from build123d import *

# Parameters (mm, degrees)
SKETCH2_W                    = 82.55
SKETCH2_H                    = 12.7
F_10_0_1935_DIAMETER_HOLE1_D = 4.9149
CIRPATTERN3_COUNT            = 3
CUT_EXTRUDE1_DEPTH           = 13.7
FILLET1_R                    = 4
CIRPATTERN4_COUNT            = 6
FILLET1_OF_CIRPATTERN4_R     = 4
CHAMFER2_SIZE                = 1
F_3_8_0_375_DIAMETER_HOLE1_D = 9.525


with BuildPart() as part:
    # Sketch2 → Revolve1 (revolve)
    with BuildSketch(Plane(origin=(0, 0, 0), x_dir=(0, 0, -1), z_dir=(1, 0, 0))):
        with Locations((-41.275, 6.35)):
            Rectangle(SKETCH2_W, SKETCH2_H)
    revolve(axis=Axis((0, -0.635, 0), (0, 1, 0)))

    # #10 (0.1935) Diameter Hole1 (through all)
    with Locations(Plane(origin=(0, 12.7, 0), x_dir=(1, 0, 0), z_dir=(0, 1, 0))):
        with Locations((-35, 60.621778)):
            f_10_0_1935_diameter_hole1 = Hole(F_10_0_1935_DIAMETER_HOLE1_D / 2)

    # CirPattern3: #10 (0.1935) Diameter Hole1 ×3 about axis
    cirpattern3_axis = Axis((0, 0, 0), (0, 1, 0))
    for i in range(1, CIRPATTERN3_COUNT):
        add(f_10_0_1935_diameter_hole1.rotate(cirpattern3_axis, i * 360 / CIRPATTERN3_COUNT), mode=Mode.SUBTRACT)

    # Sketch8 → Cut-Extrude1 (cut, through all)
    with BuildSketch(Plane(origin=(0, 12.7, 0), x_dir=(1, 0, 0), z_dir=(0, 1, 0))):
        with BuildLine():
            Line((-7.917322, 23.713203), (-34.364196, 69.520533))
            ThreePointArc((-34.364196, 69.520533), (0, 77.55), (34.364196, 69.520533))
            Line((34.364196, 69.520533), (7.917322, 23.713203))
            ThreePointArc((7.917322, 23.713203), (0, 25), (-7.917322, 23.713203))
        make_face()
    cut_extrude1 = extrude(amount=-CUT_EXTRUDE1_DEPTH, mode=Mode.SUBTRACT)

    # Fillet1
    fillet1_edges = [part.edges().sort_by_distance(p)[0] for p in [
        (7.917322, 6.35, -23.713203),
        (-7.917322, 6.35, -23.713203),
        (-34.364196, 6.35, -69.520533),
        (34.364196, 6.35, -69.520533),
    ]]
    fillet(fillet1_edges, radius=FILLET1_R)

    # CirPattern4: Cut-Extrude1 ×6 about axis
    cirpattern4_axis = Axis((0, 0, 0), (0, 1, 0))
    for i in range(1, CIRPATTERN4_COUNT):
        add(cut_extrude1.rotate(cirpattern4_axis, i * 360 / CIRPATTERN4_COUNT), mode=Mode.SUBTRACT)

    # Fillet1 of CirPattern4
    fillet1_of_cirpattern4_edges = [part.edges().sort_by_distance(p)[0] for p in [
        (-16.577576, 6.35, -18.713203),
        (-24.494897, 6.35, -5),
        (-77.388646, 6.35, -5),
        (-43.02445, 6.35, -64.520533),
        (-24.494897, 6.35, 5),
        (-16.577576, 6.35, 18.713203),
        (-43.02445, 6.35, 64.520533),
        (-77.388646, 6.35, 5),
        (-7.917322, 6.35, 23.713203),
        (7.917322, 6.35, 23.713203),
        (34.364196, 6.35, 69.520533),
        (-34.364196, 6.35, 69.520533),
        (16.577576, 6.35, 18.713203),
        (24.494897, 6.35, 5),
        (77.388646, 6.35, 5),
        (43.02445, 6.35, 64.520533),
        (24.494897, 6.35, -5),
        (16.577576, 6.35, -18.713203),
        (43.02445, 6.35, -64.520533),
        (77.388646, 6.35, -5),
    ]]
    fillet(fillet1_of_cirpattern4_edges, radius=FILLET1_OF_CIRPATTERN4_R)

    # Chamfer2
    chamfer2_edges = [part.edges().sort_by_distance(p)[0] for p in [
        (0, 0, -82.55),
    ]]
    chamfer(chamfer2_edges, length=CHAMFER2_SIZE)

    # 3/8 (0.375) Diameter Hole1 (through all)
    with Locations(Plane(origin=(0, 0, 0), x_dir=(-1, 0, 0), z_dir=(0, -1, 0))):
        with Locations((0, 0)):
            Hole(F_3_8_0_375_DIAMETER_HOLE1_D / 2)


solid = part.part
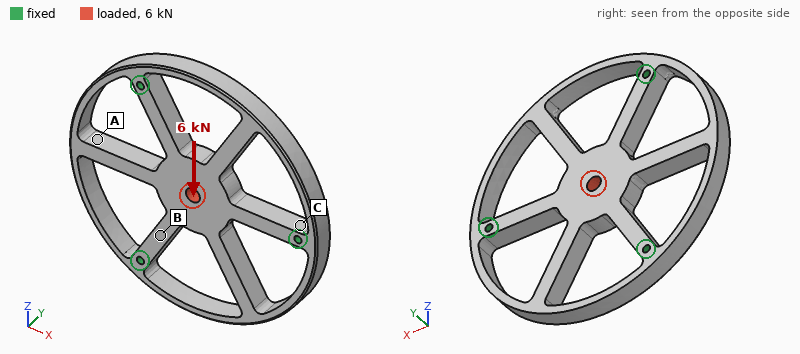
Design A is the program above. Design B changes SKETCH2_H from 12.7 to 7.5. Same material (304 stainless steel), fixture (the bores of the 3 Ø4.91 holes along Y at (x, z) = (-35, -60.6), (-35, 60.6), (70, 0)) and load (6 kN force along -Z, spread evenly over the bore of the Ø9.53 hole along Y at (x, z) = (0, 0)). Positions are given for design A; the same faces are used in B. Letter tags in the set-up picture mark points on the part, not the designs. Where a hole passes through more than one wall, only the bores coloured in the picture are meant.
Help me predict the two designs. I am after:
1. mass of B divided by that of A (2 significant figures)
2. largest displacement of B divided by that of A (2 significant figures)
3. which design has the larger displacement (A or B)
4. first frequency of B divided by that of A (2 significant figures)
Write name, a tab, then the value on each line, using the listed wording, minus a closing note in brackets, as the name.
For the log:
mass of B divided by that of A	0.59
largest displacement of B divided by that of A	1.7
which design has the larger displacement	B
first frequency of B divided by that of A	0.65
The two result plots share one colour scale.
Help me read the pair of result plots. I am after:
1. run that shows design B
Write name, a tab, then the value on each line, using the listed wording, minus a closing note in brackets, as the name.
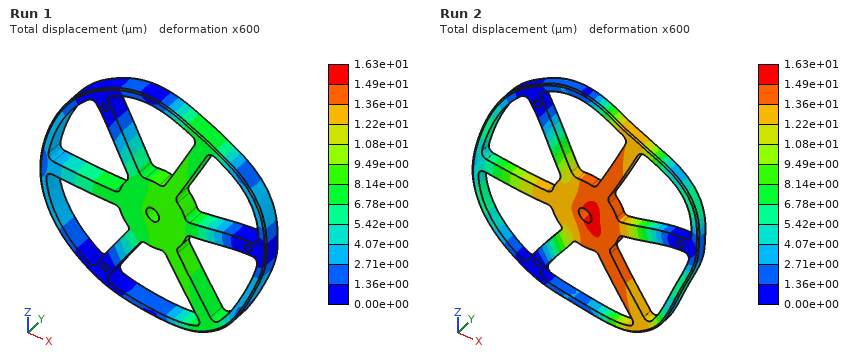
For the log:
run that shows design B	Run 2
